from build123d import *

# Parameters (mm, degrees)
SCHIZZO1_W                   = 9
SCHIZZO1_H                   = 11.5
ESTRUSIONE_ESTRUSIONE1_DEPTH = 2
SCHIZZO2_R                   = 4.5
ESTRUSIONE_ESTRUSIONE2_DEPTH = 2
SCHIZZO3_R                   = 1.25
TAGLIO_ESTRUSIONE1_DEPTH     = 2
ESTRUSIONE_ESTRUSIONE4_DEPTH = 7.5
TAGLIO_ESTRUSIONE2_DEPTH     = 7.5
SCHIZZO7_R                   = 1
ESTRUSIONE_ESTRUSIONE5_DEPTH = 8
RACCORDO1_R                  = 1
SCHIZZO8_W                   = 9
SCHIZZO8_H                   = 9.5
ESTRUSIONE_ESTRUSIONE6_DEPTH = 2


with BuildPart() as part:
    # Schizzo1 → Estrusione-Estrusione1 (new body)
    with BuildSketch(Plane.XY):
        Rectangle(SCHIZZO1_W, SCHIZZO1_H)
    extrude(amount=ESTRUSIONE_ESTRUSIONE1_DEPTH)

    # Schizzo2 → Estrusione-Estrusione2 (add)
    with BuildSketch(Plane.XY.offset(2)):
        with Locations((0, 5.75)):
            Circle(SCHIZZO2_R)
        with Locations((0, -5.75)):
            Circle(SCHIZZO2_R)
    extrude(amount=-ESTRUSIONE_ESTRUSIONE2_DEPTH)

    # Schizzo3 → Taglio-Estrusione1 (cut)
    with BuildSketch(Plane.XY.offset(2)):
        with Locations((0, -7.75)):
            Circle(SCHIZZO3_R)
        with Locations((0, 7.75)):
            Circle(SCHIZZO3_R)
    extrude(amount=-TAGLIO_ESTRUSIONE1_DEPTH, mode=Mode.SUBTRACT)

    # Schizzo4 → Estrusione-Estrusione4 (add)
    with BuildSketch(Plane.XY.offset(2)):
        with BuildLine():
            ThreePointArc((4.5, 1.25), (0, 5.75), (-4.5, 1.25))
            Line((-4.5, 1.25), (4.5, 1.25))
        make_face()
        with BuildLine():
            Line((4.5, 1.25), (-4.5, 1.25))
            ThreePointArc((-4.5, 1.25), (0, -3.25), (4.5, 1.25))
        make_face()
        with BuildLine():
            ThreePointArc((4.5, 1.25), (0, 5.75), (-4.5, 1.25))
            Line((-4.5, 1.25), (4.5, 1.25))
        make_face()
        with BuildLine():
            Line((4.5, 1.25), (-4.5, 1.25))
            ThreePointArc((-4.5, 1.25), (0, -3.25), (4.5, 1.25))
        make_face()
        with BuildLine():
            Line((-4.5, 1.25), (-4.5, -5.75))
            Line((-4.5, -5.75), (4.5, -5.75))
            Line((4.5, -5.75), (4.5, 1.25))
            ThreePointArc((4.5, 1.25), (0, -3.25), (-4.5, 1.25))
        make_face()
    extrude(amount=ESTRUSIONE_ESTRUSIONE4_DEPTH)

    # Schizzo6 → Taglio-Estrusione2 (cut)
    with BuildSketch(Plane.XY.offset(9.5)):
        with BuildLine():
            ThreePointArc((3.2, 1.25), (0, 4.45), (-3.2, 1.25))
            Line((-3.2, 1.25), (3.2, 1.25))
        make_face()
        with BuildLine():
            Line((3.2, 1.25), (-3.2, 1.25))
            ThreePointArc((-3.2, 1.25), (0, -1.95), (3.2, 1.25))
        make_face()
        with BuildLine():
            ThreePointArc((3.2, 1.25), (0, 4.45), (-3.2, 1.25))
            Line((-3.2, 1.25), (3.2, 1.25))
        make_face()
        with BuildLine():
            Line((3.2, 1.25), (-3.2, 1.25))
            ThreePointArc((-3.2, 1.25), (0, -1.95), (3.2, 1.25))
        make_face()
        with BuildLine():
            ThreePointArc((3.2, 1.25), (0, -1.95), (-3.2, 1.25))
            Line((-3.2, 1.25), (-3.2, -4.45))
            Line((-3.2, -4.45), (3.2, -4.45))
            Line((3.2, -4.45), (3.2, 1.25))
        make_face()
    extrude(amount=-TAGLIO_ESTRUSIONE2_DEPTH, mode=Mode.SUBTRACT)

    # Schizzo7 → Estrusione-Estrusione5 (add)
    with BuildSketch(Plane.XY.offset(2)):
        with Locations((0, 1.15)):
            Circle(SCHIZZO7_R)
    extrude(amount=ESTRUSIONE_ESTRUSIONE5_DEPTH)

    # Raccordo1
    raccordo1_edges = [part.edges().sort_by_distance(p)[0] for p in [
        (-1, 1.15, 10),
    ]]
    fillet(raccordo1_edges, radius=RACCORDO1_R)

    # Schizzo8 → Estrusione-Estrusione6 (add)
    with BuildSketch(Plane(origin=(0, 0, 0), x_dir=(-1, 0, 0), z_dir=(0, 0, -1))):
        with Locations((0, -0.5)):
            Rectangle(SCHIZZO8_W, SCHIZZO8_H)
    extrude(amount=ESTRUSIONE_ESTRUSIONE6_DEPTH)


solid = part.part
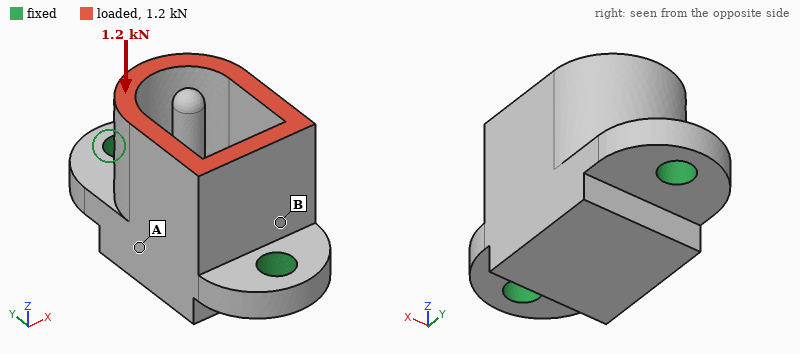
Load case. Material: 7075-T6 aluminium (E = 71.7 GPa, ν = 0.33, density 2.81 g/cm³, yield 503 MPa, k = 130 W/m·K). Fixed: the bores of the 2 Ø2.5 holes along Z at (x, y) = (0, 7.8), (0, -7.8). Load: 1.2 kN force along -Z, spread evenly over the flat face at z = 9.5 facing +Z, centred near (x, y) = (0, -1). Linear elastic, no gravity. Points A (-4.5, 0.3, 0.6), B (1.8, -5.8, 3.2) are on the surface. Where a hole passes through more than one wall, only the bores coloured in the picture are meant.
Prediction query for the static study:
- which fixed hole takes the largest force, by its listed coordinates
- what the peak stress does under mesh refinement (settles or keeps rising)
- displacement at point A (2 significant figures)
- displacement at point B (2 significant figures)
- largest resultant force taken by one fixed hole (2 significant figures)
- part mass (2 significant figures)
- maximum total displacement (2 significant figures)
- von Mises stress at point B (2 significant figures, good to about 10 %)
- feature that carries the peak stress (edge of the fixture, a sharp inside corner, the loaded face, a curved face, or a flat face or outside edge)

(0, -7.8)
keeps rising
9.8 µm
7.0 µm
650 N
2.3 g
13 µm
70 MPa
edge of the fixture
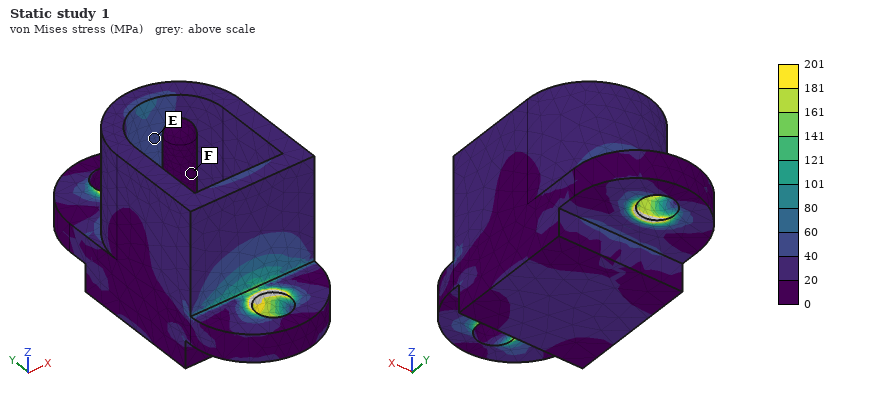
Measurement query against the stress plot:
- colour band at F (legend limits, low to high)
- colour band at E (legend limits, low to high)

0 to 20 MPa
40 to 60 MPa
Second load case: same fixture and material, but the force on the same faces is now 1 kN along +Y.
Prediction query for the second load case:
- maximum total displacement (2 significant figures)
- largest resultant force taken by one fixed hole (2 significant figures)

51 µm
850 N
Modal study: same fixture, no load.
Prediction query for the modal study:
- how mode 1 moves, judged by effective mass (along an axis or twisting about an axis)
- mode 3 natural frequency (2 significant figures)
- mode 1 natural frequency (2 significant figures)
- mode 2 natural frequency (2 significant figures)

along X
22 kHz
17 kHz
21 kHz
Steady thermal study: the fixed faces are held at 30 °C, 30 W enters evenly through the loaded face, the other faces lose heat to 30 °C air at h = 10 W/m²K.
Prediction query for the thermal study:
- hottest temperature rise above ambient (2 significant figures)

63 K
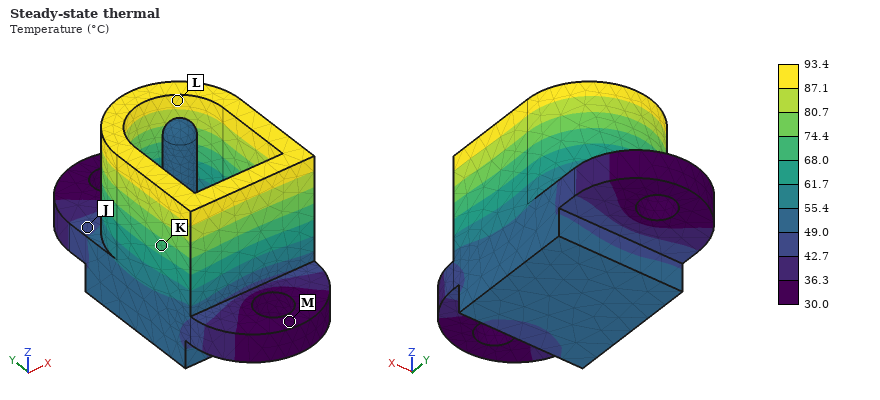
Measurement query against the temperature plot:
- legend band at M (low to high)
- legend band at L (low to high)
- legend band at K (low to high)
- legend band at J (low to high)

30.0 to 36.3 °C
87.1 to 93.4 °C
68.0 to 74.4 °C
42.7 to 49.0 °C
